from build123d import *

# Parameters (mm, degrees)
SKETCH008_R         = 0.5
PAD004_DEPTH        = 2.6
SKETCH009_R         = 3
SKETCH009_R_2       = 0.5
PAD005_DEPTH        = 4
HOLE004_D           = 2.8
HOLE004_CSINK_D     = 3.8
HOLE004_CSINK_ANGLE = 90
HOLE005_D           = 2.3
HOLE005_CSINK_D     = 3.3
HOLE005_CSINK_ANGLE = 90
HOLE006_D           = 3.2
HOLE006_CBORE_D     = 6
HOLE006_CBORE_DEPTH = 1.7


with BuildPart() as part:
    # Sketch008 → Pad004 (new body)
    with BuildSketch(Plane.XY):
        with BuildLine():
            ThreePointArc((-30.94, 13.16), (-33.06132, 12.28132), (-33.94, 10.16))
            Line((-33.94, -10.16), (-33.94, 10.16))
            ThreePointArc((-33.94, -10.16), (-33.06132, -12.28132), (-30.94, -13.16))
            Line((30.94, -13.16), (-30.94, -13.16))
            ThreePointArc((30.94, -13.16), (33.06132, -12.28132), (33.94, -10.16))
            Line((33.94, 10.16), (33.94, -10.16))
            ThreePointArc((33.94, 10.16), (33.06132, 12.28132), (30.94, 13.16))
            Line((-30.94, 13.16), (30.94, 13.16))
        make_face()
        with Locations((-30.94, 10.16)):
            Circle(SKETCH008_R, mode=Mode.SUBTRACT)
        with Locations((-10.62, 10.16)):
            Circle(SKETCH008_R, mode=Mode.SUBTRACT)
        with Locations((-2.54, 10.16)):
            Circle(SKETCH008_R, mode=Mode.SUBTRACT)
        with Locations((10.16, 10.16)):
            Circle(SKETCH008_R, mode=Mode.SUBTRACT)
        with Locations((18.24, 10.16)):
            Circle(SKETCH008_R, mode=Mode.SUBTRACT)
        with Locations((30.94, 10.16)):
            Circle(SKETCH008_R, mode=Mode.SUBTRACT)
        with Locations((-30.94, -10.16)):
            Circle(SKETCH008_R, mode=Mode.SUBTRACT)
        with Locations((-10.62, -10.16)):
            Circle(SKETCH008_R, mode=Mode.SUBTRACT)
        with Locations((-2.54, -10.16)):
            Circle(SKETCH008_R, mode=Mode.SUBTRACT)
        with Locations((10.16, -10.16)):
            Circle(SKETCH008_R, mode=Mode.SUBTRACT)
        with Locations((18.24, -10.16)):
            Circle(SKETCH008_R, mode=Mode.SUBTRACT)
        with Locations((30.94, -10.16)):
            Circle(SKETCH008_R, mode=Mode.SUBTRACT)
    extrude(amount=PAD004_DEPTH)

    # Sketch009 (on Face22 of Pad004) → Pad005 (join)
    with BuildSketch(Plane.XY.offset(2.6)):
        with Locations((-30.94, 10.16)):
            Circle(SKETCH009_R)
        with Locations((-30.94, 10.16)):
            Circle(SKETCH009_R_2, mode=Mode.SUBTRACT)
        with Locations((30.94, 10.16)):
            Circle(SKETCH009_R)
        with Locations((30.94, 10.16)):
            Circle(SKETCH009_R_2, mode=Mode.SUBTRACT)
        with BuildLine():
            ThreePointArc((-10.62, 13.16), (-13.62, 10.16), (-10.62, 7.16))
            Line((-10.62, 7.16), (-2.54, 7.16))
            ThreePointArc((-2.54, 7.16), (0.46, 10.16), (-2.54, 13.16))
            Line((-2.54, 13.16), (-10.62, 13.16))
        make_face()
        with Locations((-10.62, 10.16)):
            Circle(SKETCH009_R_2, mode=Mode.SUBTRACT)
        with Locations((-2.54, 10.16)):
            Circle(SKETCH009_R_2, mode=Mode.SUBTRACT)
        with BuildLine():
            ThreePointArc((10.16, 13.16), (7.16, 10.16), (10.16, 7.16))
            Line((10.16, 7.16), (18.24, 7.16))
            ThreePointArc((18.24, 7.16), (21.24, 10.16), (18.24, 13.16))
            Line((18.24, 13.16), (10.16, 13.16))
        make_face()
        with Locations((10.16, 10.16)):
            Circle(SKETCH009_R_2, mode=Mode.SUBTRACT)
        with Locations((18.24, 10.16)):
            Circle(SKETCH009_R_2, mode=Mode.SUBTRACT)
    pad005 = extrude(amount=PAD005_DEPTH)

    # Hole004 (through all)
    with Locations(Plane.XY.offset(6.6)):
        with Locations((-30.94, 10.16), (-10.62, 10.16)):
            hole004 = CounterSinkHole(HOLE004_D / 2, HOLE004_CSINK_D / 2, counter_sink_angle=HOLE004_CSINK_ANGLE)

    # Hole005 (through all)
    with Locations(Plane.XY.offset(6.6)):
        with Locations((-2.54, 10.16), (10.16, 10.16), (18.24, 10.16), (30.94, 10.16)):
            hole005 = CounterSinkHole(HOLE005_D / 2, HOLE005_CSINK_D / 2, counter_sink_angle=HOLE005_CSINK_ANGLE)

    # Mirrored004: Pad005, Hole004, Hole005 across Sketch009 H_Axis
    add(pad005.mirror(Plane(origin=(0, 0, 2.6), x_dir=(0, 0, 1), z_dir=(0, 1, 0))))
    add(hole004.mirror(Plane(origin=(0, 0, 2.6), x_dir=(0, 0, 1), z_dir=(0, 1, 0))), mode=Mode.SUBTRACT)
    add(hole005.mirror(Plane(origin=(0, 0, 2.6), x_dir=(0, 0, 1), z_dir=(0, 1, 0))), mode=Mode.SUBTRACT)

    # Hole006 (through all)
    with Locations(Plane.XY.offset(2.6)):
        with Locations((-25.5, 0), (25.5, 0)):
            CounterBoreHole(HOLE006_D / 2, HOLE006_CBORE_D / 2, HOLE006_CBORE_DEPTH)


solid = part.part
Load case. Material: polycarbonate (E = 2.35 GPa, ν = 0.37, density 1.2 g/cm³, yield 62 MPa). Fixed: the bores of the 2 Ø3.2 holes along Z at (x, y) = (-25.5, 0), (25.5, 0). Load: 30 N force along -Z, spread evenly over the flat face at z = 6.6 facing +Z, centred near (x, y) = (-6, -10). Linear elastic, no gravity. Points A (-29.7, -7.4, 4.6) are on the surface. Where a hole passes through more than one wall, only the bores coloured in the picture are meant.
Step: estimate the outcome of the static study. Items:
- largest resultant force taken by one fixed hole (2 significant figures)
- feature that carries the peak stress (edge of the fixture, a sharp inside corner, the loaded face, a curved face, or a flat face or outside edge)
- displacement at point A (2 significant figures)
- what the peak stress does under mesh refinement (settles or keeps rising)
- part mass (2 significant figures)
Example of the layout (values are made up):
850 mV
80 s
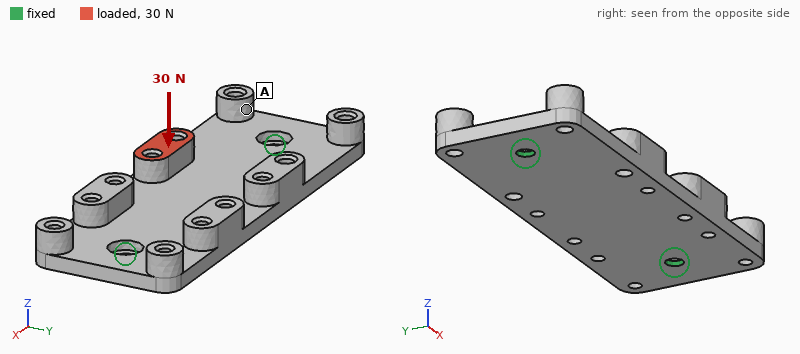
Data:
47 N
edge of the fixture
0.21 mm
keeps rising
7.0 g
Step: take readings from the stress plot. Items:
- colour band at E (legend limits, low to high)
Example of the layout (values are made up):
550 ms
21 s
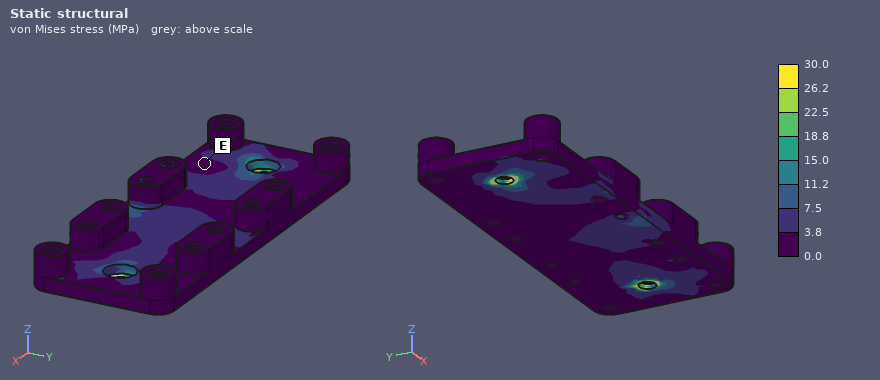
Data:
0.0 to 3.8 MPa
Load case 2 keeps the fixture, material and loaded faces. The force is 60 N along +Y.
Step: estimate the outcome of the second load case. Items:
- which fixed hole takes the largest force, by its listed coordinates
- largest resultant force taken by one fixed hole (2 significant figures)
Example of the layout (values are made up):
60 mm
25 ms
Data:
(-25.5, 0)
38 N
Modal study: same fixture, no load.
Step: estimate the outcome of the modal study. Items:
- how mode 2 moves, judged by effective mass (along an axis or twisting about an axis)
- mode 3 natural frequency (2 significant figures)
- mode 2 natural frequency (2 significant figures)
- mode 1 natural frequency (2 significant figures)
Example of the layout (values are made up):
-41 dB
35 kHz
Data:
along Z
1600 Hz
940 Hz
720 Hz
